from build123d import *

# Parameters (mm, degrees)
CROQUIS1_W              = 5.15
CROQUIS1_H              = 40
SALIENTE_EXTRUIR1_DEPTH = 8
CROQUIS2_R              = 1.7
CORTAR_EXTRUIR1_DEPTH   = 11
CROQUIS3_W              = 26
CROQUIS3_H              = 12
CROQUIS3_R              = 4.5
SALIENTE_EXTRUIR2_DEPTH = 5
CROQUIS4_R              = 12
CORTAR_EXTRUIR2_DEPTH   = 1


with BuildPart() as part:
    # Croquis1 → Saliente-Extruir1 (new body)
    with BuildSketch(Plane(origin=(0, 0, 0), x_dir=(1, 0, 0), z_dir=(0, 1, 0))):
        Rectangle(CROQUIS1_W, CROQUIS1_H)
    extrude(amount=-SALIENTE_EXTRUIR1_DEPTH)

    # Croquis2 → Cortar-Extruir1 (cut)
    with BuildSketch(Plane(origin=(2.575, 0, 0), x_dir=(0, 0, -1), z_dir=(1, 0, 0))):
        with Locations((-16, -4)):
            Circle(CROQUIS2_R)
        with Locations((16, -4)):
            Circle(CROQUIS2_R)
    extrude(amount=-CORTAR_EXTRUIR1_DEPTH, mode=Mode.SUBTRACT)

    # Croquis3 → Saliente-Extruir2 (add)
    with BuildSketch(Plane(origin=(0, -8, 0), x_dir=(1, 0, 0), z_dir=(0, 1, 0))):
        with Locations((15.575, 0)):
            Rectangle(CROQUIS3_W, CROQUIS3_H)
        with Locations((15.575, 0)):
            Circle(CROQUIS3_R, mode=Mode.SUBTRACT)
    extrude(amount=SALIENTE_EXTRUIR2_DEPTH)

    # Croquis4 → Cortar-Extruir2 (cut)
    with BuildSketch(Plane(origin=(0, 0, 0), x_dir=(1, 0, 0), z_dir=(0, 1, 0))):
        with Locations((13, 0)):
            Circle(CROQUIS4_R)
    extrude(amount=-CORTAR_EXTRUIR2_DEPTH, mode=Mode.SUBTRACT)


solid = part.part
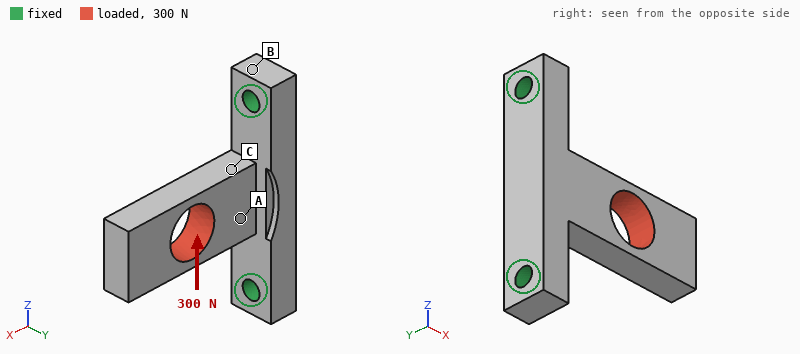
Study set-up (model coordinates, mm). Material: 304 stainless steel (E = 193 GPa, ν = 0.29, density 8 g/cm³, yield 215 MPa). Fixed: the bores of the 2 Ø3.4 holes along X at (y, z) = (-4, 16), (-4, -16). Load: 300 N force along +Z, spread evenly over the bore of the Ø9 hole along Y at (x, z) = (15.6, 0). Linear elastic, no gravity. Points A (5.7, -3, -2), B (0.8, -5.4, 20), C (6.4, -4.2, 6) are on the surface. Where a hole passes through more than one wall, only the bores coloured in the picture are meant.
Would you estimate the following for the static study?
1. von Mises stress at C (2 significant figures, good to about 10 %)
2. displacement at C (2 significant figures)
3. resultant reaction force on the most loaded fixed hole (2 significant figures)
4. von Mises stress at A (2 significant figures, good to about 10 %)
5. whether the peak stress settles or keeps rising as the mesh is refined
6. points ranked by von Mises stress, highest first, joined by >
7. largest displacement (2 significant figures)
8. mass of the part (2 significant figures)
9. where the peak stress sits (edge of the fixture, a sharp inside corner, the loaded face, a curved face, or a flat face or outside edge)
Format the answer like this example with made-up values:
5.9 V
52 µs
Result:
26 MPa
3.2 µm
260 N
16 MPa
keeps rising
C > A > B
19 µm
22 g
a sharp inside corner
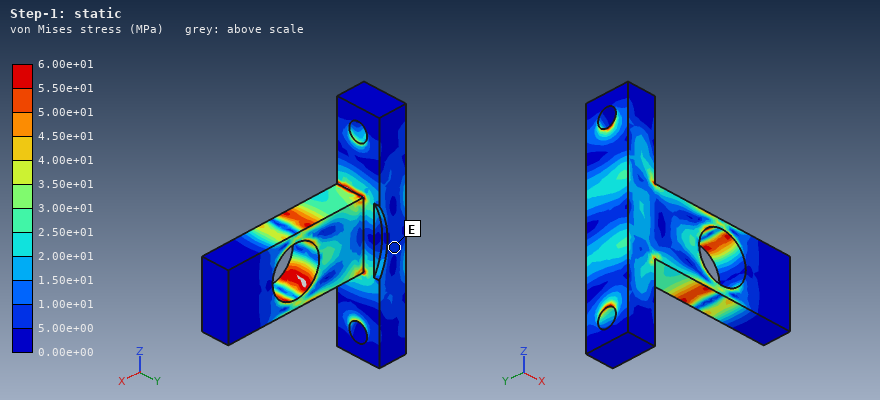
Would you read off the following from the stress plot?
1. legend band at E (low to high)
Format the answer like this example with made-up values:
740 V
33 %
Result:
5.00e+00 to 1.00e+01 MPa
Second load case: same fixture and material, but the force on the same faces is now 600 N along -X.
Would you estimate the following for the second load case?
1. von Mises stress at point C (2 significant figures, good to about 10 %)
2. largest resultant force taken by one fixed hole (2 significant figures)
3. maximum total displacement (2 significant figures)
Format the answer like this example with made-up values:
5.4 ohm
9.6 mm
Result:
17 MPa
310 N
10 µm
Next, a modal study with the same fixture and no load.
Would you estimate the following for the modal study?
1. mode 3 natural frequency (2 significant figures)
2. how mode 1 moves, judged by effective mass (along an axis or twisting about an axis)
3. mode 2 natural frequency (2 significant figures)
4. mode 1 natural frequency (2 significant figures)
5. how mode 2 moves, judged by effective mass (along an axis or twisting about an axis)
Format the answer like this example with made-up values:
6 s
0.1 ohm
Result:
15 kHz
along Y
7000 Hz
3400 Hz
along Z
